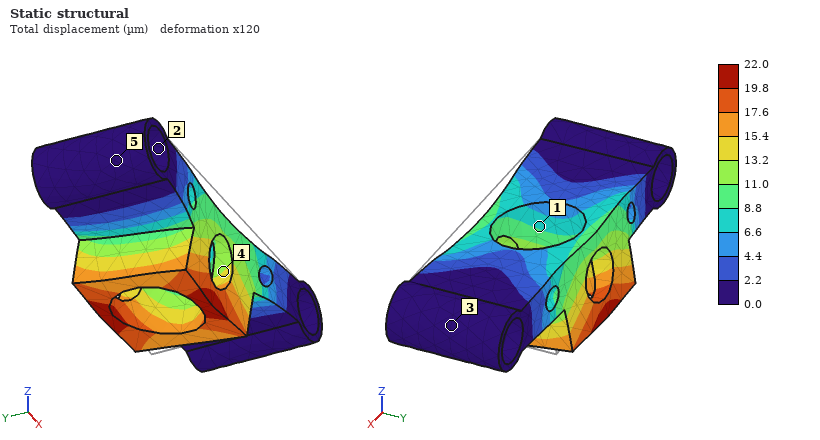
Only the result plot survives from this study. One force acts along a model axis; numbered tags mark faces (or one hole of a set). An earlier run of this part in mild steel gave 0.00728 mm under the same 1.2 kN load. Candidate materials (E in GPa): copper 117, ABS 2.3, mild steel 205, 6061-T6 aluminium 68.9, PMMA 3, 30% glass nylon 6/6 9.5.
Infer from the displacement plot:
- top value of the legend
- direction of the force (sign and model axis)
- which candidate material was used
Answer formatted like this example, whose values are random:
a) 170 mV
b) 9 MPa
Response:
a) 22.0 µm
b) +Y
c) 6061-T6 aluminium
